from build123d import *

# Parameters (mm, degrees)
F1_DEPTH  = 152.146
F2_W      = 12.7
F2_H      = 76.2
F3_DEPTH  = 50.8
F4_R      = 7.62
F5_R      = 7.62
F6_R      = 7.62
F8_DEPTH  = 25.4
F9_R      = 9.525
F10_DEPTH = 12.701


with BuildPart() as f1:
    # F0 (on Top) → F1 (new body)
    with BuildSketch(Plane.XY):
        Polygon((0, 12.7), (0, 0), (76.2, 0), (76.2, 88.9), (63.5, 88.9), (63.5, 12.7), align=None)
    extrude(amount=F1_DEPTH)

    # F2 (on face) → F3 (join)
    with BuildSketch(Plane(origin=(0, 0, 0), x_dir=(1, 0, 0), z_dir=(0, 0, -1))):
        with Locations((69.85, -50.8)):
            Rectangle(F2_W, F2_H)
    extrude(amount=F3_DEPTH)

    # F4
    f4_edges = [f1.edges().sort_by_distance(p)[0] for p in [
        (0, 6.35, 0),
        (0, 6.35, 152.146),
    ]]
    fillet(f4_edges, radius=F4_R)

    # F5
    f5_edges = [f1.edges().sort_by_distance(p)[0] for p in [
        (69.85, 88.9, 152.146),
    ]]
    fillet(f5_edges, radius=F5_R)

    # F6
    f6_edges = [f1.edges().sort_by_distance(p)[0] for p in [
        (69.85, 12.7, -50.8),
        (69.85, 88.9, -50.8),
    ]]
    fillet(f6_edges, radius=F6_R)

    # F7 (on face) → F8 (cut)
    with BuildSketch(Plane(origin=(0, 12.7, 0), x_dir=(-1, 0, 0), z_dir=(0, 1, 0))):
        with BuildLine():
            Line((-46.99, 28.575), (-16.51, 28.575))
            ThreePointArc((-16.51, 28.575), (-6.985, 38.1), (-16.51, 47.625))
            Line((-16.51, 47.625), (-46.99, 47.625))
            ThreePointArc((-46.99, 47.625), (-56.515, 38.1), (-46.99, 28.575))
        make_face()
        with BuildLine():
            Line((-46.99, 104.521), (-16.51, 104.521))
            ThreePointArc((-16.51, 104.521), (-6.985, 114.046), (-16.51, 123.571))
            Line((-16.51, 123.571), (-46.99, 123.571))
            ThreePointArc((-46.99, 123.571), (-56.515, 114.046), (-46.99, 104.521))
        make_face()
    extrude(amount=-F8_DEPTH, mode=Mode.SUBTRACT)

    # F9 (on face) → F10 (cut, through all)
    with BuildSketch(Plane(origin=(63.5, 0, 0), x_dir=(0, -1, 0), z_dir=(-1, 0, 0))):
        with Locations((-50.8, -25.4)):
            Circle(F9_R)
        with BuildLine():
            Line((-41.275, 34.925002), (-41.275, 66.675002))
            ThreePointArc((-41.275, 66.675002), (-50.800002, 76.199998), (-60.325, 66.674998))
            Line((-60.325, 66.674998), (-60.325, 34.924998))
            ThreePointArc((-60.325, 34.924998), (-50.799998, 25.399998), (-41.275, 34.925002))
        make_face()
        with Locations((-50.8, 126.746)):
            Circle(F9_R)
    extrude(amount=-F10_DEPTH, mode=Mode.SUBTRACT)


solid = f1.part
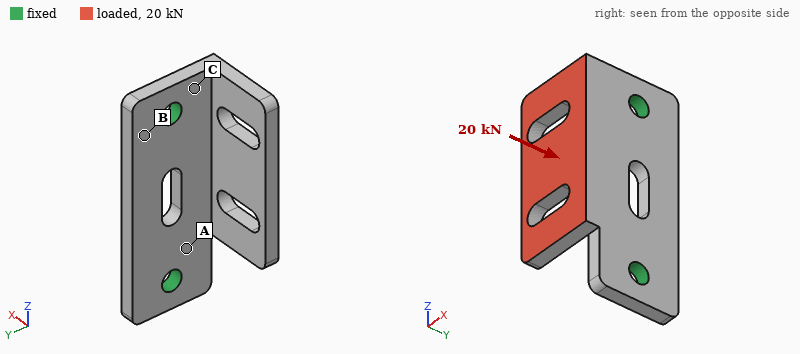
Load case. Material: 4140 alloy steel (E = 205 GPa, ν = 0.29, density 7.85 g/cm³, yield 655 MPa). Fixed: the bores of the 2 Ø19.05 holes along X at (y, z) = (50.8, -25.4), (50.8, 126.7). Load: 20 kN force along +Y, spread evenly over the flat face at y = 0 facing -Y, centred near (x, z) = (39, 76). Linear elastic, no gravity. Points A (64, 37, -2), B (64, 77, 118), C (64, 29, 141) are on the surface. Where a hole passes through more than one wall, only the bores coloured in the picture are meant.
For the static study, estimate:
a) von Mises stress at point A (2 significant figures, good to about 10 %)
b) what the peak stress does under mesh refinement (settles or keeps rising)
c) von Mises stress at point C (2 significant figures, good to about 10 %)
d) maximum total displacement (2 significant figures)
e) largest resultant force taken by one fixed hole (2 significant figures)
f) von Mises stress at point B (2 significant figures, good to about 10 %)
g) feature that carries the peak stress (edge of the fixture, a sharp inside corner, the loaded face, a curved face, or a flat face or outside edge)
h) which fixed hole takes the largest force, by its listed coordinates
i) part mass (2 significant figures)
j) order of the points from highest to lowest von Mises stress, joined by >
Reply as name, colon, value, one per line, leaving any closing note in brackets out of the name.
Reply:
von Mises stress at point A: 130 MPa
what the peak stress does under mesh refinement: keeps rising
von Mises stress at point C: 180 MPa
maximum total displacement: 0.55 mm
largest resultant force taken by one fixed hole: 14 kN
von Mises stress at point B: 35 MPa
feature that carries the peak stress: edge of the fixture
which fixed hole takes the largest force, by its listed coordinates: (50.8, 126.7)
part mass: 2.4 kg
order of the points from highest to lowest von Mises stress, joined by >: C > A > B
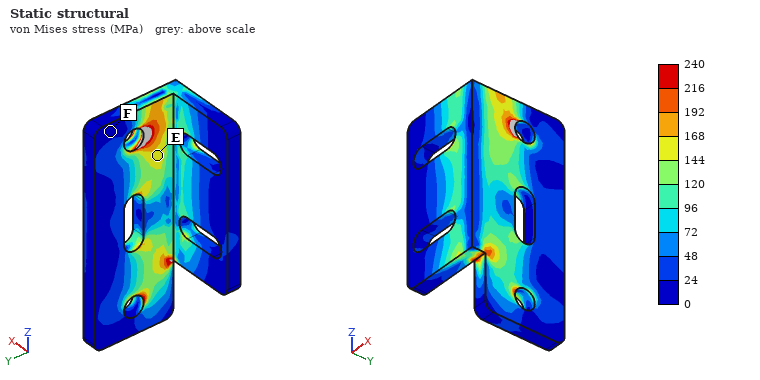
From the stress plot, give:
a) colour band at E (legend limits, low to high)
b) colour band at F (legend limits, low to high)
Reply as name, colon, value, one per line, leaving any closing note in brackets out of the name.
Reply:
colour band at E: 144 to 168 MPa
colour band at F: 0 to 24 MPa
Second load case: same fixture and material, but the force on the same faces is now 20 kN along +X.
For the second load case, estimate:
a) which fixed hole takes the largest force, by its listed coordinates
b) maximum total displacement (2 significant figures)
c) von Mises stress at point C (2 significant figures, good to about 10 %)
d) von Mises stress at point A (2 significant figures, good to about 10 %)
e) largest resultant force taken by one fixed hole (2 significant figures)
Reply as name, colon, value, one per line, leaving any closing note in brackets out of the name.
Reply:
which fixed hole takes the largest force, by its listed coordinates: (50.8, 126.7)
maximum total displacement: 0.45 mm
von Mises stress at point C: 180 MPa
von Mises stress at point A: 140 MPa
largest resultant force taken by one fixed hole: 13 kN
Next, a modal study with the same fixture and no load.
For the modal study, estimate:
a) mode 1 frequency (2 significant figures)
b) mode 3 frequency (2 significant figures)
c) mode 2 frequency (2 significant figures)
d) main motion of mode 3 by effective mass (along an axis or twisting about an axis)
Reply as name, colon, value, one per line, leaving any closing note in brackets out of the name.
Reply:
mode 1 frequency: 1100 Hz
mode 3 frequency: 2500 Hz
mode 2 frequency: 2000 Hz
main motion of mode 3 by effective mass: along X
